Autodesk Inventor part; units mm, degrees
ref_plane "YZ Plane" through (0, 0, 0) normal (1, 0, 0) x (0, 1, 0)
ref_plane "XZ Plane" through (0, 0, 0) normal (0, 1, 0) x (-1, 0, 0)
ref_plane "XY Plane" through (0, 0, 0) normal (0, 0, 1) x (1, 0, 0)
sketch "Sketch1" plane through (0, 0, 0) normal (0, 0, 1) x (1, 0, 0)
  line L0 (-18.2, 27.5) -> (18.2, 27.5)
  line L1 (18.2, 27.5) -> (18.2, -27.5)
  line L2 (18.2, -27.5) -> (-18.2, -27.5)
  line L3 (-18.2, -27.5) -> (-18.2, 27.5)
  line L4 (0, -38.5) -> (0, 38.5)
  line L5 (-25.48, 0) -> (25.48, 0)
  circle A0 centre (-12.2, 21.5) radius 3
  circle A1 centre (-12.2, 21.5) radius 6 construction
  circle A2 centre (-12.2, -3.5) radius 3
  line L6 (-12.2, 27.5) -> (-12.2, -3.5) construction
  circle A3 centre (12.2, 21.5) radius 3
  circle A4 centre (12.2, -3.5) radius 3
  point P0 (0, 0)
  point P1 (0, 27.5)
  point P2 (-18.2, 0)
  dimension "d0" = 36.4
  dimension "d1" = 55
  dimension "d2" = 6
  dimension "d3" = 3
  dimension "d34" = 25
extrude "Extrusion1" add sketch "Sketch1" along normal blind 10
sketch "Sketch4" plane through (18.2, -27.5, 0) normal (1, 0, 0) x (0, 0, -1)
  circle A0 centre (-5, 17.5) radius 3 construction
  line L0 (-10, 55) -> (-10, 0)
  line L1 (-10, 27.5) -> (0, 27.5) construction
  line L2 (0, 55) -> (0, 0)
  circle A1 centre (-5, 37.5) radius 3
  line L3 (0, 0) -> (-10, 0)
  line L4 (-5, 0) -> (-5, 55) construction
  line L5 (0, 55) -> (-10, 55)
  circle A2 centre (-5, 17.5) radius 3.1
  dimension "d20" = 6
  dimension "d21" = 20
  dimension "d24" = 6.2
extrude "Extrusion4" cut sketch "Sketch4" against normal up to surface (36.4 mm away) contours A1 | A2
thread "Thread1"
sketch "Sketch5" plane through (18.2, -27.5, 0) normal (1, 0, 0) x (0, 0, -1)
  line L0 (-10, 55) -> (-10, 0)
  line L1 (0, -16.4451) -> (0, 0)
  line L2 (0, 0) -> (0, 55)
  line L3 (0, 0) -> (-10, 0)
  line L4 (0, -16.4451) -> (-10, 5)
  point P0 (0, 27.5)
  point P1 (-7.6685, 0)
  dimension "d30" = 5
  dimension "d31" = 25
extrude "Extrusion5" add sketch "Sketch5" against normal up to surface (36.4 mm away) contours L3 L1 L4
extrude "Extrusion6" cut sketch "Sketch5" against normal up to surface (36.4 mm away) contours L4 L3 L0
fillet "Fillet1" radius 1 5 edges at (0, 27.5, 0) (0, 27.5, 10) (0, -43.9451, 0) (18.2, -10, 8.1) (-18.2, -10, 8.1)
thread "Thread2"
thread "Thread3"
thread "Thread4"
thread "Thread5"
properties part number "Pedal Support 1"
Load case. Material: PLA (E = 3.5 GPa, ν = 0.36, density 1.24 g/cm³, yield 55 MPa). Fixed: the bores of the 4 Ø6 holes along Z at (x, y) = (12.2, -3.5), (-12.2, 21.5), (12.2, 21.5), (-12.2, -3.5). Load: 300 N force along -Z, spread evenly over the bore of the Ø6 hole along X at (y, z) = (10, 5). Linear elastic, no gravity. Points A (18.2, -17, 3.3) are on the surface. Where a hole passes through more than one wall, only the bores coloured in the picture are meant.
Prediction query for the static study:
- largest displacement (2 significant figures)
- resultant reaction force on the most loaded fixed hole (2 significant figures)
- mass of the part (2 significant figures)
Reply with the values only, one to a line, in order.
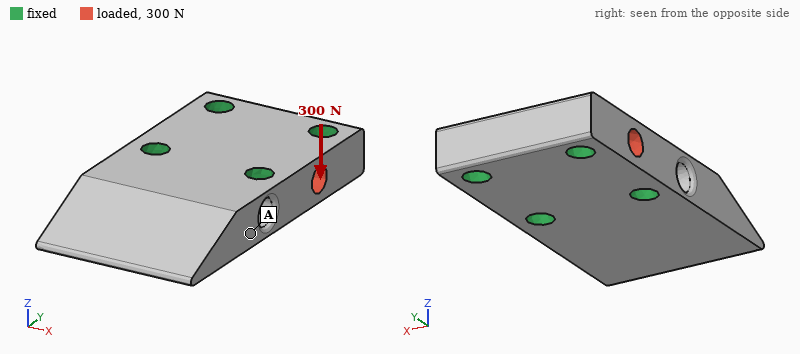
7.5 µm
80 N
23 g
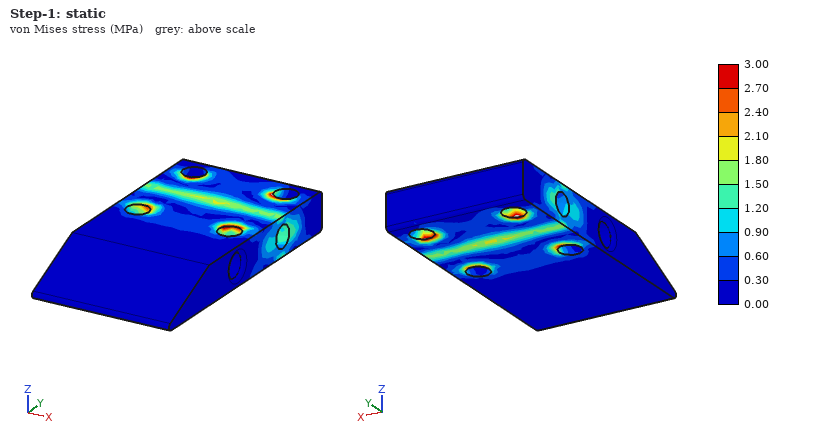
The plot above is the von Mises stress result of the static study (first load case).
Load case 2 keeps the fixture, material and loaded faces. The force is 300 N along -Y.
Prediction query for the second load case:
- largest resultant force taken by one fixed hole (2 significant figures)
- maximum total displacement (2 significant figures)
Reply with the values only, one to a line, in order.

79 N
2.1 µm
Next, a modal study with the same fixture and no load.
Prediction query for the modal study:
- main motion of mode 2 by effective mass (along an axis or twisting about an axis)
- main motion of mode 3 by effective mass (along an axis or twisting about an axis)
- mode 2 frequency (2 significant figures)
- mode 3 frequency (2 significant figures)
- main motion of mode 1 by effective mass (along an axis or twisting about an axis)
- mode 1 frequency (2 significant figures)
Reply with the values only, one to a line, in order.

twisting about Y
along X
4100 Hz
5000 Hz
along Z
2400 Hz
